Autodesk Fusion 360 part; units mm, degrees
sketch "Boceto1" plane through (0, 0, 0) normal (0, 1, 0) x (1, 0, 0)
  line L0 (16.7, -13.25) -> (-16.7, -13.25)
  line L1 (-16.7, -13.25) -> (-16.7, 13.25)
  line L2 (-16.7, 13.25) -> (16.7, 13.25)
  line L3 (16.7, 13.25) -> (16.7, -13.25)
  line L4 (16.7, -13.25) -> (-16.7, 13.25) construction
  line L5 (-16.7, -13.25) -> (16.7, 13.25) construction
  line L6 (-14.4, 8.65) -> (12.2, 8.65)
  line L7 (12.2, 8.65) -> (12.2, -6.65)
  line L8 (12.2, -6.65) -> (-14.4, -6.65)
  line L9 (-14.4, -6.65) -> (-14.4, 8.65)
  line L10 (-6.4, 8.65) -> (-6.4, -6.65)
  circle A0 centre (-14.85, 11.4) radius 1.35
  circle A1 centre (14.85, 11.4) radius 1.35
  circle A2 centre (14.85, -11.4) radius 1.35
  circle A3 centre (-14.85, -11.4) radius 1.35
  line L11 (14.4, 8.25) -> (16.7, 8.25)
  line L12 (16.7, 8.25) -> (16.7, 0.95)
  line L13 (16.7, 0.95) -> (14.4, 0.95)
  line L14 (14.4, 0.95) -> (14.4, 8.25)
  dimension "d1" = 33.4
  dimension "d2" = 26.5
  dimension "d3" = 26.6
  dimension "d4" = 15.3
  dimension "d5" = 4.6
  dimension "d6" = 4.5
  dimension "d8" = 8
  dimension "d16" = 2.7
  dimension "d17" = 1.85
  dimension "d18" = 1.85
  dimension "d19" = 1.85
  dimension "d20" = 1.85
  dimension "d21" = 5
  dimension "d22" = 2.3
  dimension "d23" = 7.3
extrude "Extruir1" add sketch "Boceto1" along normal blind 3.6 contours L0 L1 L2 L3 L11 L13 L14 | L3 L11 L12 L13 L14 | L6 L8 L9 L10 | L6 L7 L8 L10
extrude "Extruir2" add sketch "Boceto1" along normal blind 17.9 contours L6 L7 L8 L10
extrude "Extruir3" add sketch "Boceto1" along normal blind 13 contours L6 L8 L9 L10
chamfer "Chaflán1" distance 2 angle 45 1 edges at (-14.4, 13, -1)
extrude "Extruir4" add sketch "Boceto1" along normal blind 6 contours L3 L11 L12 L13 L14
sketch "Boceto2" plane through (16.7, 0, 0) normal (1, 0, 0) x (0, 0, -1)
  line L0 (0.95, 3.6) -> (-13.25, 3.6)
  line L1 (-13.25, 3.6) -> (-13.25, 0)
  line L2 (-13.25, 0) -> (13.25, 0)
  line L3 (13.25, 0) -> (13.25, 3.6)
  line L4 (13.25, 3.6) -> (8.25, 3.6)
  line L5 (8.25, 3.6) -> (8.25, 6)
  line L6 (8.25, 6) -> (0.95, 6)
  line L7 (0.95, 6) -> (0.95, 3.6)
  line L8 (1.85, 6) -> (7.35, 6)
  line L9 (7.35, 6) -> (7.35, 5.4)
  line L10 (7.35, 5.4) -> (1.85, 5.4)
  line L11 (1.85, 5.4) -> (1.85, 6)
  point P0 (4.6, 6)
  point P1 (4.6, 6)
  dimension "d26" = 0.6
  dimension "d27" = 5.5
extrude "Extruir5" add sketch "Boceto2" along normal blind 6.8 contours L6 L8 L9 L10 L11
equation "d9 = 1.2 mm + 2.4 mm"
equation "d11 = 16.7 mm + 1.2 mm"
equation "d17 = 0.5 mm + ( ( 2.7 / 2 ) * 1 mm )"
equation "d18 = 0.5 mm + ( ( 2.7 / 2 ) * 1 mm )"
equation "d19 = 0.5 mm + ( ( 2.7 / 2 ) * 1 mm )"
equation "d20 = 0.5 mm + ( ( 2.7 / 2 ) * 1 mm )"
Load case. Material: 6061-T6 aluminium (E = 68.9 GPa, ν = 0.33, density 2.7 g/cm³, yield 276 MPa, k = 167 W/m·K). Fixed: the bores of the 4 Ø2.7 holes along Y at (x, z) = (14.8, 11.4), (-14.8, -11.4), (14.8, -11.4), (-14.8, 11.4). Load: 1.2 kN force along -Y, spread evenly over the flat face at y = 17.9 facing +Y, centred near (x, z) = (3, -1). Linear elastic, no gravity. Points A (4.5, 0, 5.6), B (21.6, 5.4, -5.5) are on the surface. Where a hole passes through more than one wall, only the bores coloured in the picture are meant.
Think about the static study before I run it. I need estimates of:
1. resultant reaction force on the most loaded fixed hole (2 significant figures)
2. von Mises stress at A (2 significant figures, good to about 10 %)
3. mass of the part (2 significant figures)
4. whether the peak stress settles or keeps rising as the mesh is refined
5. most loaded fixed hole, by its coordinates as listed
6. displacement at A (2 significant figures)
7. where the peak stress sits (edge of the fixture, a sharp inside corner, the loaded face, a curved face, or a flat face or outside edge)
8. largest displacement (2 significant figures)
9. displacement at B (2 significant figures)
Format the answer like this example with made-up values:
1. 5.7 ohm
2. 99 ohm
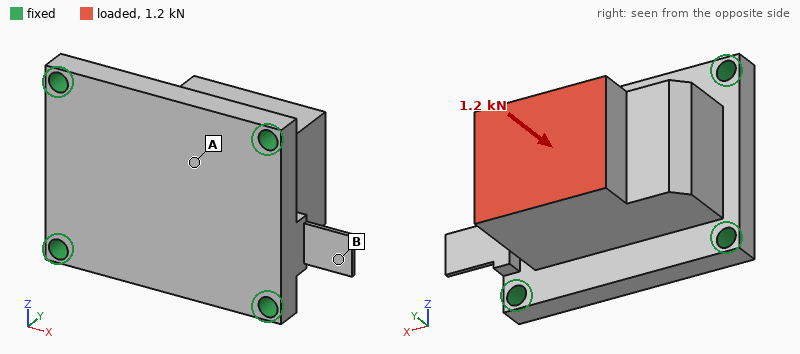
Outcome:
1. 430 N
2. 14 MPa
3. 23 g
4. keeps rising
5. (14.8, -11.4)
6. 8.1 µm
7. edge of the fixture
8. 10 µm
9. 2.6 µm
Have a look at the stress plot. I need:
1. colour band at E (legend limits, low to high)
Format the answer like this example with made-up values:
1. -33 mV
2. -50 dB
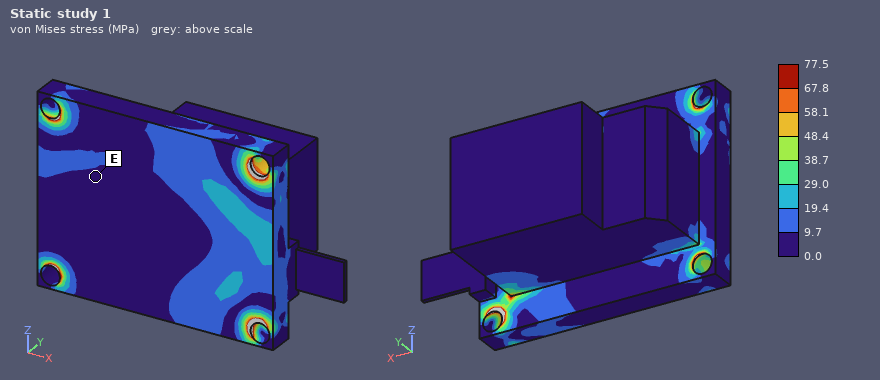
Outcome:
1. 0.0 to 9.7 MPa
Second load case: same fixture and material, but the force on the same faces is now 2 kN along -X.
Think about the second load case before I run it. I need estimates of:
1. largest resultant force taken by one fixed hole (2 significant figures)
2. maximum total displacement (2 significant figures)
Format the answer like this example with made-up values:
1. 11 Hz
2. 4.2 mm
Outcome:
1. 1.0 kN
2. 27 µm
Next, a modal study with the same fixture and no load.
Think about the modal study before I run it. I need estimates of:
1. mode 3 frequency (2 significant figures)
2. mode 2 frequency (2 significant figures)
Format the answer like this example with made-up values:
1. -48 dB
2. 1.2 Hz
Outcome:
1. 16 kHz
2. 14 kHz
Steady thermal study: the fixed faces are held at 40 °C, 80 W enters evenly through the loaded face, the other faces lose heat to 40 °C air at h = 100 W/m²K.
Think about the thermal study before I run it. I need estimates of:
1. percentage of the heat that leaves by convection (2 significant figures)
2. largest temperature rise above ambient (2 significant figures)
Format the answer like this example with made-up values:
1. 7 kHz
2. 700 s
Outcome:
1. 8.8 %
2. 48 K
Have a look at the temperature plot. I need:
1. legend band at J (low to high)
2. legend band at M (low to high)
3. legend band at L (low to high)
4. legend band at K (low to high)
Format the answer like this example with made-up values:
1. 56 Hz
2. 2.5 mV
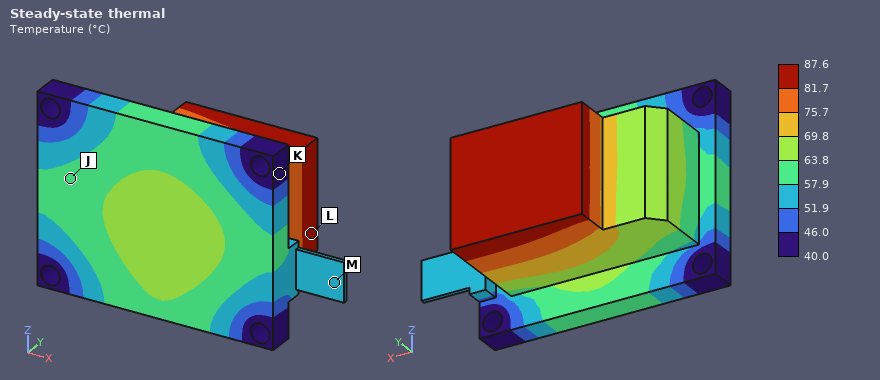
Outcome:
1. 57.9 to 63.8 °C
2. 51.9 to 57.9 °C
3. 81.7 to 87.6 °C
4. 40.0 to 46.0 °C
